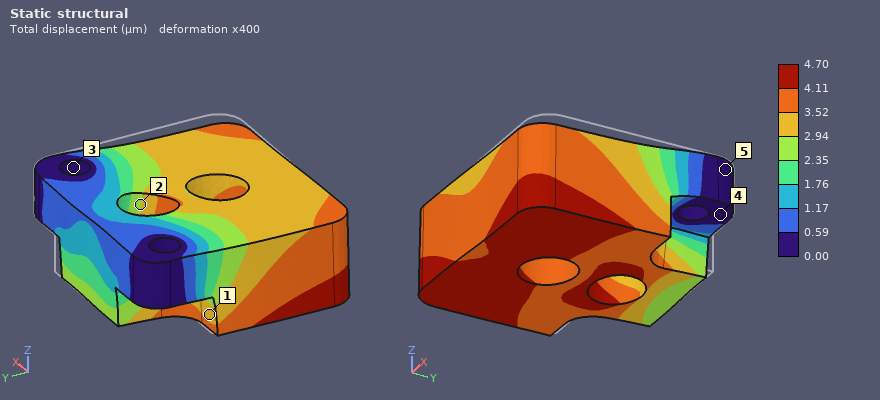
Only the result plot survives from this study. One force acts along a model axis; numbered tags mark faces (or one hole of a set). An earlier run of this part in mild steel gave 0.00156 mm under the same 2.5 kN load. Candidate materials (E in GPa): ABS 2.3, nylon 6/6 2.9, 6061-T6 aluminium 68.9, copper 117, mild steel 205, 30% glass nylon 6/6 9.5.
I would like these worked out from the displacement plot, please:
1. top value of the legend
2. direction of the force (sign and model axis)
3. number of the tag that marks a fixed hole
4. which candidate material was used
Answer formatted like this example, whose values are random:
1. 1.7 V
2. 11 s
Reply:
1. 4.70 µm
2. -X
3. 3
4. 6061-T6 aluminium
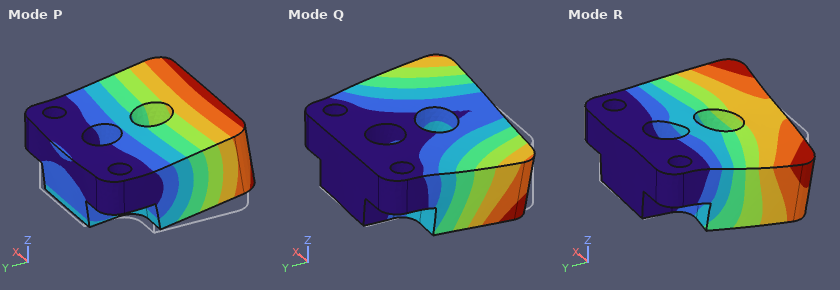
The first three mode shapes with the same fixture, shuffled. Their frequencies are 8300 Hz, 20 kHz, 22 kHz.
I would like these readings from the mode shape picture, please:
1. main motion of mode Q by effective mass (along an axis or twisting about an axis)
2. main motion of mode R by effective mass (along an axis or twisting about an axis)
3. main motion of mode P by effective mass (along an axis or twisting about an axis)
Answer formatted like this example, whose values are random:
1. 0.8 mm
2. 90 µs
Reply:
1. along X
2. along X
3. along Z
